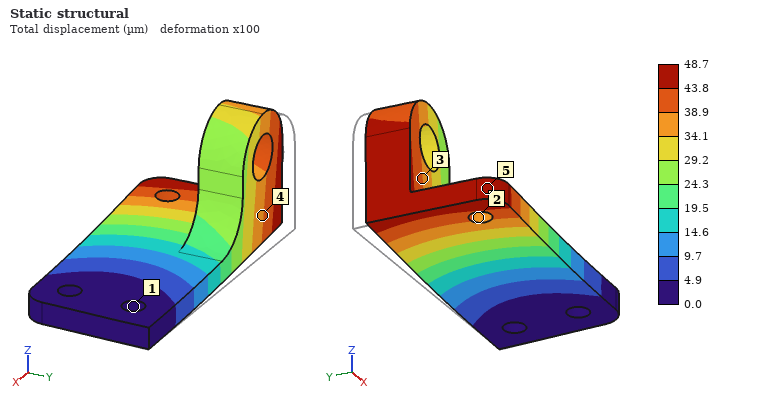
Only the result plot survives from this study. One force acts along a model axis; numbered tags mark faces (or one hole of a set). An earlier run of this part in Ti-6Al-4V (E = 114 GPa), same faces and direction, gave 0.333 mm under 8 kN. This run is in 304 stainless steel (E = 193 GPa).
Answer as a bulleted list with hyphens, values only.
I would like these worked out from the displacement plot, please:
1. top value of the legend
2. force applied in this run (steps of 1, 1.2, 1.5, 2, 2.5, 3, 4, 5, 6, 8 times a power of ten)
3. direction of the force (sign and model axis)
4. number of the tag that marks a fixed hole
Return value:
- 48.7 µm
- 2 kN
- -Y
- 1
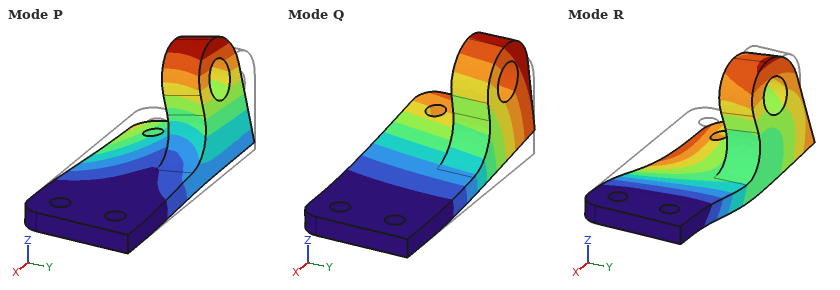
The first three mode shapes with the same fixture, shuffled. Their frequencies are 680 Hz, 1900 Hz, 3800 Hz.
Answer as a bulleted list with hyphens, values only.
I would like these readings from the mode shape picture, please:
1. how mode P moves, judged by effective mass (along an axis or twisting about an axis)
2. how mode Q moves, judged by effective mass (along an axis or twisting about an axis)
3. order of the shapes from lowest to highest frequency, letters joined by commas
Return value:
- along Y
- along Z
- Q, P, R
